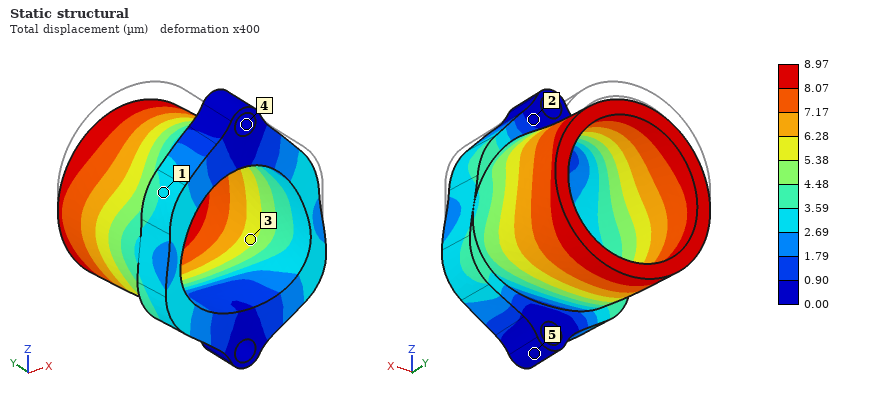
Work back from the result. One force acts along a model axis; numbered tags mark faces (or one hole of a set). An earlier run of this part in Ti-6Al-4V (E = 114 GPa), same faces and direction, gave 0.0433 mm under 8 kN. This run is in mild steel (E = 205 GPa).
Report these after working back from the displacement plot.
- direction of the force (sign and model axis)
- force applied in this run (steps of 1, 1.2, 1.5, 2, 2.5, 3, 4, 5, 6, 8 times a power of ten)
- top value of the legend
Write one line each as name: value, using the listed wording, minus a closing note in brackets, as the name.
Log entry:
direction of the force: -Z
force applied in this run: 3 kN
top value of the legend: 8.97 µm
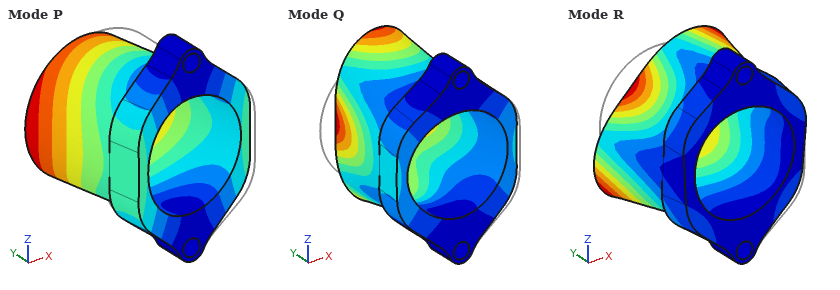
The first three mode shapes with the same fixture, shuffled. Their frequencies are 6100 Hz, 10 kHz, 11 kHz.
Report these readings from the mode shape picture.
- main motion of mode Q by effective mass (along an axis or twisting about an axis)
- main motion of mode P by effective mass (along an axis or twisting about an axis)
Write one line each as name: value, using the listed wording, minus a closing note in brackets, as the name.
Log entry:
main motion of mode Q by effective mass: along Y
main motion of mode P by effective mass: along X
